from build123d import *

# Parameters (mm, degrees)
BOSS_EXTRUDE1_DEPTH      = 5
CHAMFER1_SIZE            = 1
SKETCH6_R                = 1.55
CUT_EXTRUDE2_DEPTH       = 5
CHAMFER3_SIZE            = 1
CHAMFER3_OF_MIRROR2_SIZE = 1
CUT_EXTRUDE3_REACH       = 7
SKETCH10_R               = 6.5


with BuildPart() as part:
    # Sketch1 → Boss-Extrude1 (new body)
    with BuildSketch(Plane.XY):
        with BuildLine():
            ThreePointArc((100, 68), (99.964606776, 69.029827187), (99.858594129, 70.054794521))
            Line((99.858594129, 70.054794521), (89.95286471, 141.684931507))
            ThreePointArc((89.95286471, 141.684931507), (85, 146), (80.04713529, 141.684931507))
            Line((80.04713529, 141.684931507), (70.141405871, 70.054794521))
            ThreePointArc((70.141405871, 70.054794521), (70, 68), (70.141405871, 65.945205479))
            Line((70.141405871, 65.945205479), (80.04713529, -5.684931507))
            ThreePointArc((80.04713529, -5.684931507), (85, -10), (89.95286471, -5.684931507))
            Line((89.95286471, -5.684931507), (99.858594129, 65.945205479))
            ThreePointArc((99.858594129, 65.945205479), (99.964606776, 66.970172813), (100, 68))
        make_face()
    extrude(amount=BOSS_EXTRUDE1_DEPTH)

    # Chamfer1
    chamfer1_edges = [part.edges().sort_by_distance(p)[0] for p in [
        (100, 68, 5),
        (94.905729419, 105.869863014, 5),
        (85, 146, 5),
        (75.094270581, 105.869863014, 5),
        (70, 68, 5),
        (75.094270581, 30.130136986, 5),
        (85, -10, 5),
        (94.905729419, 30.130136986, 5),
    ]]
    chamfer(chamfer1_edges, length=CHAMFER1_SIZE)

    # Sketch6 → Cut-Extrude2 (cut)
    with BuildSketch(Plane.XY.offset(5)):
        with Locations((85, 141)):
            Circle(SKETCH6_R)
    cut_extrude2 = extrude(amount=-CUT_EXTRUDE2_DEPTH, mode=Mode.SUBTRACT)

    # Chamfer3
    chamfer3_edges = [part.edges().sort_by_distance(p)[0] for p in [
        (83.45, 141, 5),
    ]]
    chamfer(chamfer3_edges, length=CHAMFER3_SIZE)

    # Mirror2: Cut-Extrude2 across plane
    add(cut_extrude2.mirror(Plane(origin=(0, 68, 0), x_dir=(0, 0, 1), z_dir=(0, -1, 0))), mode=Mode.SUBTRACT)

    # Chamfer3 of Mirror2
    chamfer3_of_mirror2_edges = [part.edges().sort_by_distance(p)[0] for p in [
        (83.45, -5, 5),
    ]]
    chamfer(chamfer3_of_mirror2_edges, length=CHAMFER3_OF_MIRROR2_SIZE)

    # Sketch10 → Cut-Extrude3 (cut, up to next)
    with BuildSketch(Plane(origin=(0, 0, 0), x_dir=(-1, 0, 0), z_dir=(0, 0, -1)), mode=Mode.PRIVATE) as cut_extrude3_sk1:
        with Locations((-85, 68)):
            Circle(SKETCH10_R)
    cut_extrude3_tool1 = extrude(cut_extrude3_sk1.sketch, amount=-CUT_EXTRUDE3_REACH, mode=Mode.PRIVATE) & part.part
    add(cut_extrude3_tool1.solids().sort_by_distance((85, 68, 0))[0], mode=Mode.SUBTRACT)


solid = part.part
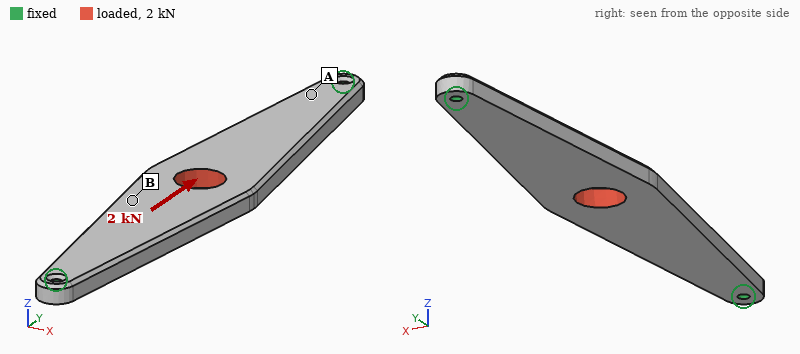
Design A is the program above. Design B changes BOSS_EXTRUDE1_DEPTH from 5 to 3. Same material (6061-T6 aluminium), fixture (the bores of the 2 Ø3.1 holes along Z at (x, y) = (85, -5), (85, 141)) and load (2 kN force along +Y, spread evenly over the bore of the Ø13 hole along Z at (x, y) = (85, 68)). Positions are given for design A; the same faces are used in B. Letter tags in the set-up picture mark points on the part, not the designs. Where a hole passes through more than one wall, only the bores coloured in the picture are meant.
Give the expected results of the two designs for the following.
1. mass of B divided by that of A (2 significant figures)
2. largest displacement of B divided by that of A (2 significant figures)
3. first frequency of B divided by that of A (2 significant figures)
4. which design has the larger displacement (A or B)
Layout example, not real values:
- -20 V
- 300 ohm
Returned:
- 0.60
- 1.7
- 0.61
- B
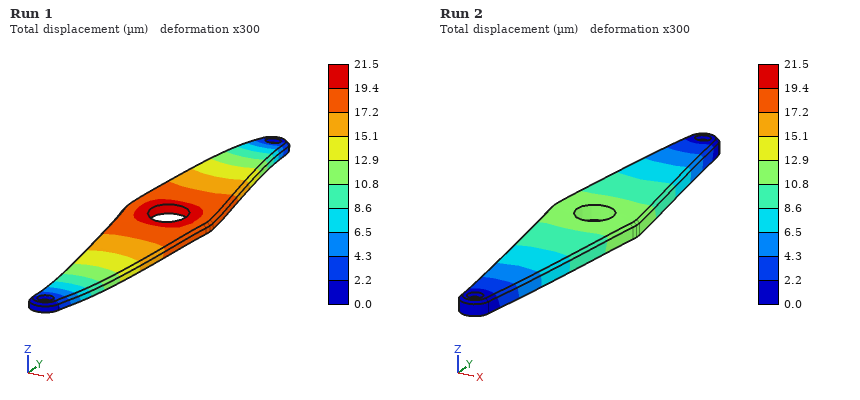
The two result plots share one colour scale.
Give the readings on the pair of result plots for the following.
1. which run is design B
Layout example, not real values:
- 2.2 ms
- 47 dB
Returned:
- Run 1
